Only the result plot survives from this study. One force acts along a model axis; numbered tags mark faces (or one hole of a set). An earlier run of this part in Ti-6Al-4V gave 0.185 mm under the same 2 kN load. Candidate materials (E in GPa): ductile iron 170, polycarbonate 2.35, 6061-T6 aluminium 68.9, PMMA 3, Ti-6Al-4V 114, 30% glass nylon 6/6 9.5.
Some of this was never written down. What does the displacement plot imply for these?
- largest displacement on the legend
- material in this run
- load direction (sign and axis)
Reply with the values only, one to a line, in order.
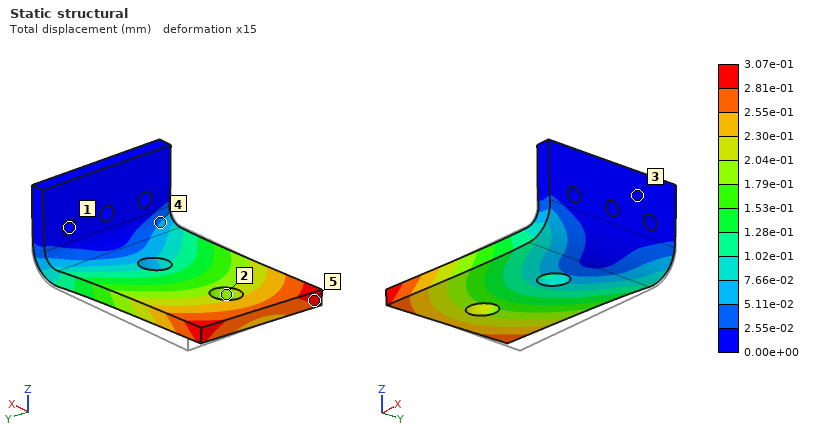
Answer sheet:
3.07e-01 mm
6061-T6 aluminium
-Y
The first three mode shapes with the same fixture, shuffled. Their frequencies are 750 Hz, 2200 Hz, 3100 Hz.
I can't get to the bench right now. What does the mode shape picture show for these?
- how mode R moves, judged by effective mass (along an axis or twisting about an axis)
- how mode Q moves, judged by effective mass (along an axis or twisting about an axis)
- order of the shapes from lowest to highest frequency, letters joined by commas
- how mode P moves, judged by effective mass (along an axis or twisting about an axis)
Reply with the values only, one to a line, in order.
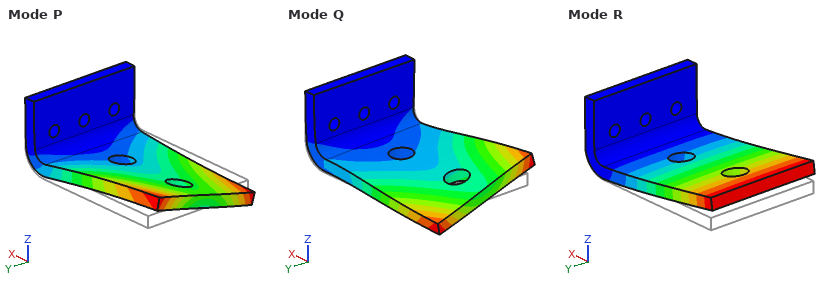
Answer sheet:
along Z
along Y
R, P, Q
along Y
